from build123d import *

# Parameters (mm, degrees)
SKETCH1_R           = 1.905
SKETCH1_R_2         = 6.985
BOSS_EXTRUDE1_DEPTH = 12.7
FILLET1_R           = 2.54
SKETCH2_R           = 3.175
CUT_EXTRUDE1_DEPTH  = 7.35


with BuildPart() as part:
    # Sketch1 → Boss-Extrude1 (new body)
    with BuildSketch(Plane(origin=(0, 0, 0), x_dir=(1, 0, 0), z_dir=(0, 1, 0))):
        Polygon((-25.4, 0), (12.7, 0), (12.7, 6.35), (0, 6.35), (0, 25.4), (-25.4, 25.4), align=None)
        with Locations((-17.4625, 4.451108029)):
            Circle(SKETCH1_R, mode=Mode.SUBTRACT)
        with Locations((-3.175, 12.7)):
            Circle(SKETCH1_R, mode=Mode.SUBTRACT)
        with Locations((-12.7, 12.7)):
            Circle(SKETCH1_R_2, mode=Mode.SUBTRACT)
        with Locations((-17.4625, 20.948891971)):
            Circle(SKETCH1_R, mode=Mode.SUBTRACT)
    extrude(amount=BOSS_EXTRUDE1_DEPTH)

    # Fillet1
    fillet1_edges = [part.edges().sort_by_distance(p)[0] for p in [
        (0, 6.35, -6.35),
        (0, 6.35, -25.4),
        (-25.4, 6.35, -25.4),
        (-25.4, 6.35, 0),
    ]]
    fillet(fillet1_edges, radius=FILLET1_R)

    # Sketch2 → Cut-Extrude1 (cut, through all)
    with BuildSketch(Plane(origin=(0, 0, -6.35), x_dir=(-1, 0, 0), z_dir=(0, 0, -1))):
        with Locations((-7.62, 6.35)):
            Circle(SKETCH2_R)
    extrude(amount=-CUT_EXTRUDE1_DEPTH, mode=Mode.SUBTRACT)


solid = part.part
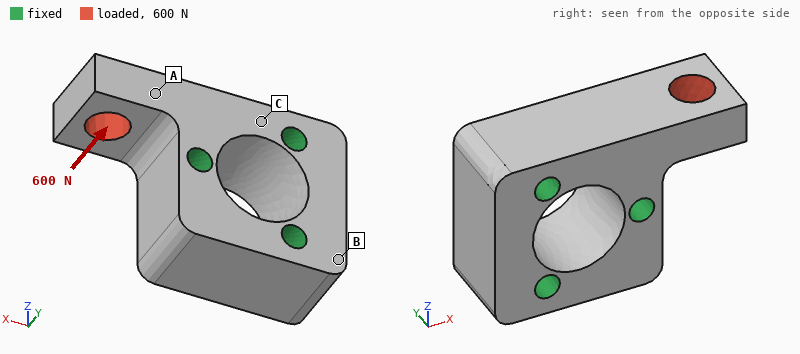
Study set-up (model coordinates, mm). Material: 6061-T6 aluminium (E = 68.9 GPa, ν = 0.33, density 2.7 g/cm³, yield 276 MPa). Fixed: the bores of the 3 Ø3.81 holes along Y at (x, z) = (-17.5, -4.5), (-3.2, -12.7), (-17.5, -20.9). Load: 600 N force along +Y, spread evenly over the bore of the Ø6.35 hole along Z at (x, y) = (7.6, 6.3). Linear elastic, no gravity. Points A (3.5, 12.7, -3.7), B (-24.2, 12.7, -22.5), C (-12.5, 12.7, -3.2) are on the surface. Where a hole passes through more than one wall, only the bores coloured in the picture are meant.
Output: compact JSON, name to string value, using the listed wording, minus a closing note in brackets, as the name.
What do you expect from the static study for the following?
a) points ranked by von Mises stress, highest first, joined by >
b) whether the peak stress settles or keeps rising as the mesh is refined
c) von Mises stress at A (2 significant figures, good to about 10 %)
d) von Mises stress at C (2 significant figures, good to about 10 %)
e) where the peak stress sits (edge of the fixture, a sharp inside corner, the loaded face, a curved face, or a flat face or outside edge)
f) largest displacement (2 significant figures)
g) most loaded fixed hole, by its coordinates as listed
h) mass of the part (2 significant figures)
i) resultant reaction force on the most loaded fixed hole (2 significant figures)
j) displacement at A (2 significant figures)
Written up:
{"points ranked by von Mises stress, highest first, joined by >": "A > C > B", "whether the peak stress settles or keeps rising as the mesh is refined": "keeps rising", "von Mises stress at A": "27 MPa", "von Mises stress at C": "20 MPa", "where the peak stress sits": "edge of the fixture", "largest displacement": "26 µm", "most loaded fixed hole, by its coordinates as listed": "(-3.2, -12.7)", "mass of the part": "18 g", "resultant reaction force on the most loaded fixed hole": "670 N", "displacement at A": "11 µm"}
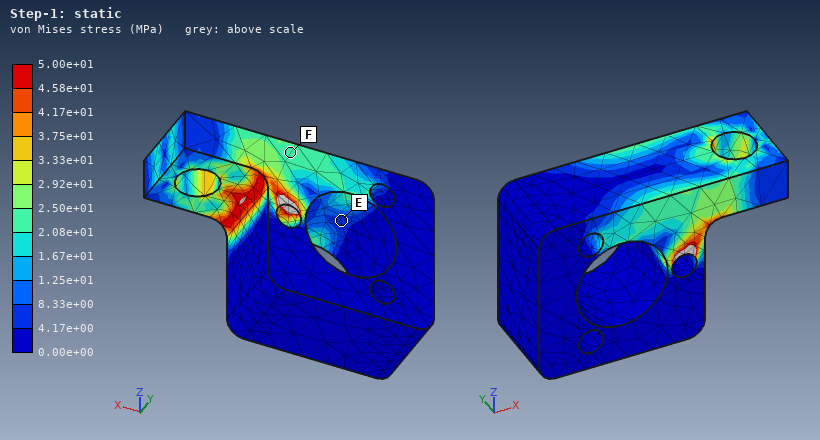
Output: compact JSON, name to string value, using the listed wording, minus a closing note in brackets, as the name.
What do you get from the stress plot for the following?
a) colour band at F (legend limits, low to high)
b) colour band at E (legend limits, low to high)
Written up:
{"colour band at F": "2.08e+01 to 2.50e+01 MPa", "colour band at E": "4.17e+00 to 8.33e+00 MPa"}
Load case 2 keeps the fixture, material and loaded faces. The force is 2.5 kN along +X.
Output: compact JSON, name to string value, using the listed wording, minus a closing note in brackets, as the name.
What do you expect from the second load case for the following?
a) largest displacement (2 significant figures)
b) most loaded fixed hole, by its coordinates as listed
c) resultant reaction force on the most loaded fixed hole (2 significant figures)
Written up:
{"largest displacement": "23 µm", "most loaded fixed hole, by its coordinates as listed": "(-17.5, -4.5)", "resultant reaction force on the most loaded fixed hole": "1.9 kN"}
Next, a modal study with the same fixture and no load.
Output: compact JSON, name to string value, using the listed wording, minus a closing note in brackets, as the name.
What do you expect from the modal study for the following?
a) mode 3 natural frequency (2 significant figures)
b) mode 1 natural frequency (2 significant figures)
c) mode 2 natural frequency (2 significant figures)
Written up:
{"mode 3 natural frequency": "35 kHz", "mode 1 natural frequency": "20 kHz", "mode 2 natural frequency": "21 kHz"}
